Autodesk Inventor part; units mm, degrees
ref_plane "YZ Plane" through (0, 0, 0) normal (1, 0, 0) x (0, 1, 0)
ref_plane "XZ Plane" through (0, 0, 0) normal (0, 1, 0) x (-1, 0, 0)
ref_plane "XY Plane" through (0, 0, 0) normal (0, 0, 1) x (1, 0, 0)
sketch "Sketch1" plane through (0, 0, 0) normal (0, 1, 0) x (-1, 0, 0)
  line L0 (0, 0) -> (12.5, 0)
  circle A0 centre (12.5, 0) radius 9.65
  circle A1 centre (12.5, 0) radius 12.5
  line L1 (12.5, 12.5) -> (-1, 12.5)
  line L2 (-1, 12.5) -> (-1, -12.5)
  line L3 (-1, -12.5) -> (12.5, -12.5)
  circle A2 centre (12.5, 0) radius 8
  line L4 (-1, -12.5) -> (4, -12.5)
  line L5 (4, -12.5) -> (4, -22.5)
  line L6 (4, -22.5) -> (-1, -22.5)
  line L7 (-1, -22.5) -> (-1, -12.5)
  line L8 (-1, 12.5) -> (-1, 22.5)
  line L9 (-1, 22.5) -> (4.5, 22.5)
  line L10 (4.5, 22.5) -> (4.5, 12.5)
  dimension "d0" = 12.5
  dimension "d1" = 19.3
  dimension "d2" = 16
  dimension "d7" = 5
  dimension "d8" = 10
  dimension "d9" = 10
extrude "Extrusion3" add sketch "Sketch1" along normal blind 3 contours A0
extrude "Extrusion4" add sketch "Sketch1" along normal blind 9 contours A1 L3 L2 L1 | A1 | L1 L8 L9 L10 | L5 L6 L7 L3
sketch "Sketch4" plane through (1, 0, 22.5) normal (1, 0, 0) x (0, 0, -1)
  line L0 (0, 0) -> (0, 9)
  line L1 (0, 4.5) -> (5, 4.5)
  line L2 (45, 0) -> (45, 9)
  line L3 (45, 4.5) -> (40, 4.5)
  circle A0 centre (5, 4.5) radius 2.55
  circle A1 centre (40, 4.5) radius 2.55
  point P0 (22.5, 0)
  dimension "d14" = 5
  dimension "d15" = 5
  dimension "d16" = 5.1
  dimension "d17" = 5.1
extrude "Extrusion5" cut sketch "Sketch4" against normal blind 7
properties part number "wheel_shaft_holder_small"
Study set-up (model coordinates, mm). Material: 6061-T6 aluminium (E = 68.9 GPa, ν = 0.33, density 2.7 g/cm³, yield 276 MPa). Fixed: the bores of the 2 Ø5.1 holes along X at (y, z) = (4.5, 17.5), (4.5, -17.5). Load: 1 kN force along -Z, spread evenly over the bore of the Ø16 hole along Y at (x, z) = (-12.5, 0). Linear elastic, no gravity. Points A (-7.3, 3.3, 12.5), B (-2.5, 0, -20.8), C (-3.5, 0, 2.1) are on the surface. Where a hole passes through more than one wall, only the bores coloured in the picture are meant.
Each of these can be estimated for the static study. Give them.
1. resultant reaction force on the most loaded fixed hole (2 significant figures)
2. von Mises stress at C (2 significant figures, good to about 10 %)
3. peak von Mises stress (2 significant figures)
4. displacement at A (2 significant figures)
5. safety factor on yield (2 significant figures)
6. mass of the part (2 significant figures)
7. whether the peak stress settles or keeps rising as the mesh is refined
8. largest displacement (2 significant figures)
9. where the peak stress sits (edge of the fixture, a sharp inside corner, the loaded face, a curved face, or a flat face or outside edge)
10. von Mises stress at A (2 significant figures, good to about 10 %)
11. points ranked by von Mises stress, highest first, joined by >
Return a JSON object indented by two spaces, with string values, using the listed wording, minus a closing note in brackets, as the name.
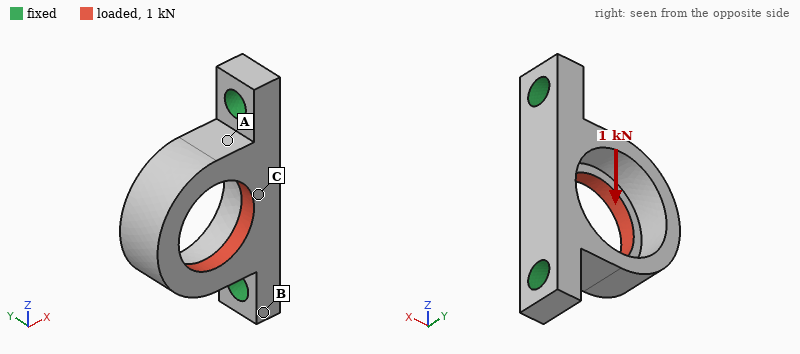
{
  "resultant reaction force on the most loaded fixed hole": "640 N",
  "von Mises stress at C": "28 MPa",
  "peak von Mises stress": "82 MPa",
  "displacement at A": "6.3 µm",
  "safety factor on yield": "3.4",
  "mass of the part": "9.8 g",
  "whether the peak stress settles or keeps rising as the mesh is refined": "settles",
  "largest displacement": "35 µm",
  "where the peak stress sits": "the loaded face",
  "von Mises stress at A": "48 MPa",
  "points ranked by von Mises stress, highest first, joined by >": "A > C > B"
}
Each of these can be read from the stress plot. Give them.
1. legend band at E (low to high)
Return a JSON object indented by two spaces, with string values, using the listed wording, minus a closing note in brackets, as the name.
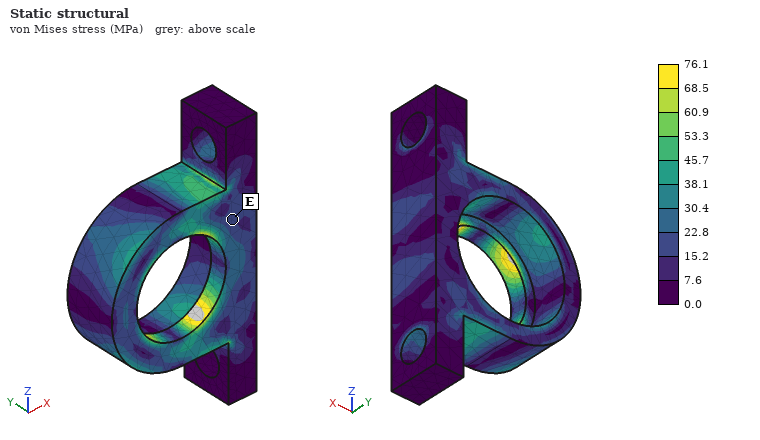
{
  "legend band at E": "15.2 to 22.8 MPa"
}
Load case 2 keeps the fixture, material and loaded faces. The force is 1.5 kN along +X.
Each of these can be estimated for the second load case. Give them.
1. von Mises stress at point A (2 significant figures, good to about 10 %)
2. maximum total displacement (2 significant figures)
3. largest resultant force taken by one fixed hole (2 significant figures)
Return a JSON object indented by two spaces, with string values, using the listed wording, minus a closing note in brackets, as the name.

{
  "von Mises stress at point A": "44 MPa",
  "maximum total displacement": "54 µm",
  "largest resultant force taken by one fixed hole": "770 N"
}
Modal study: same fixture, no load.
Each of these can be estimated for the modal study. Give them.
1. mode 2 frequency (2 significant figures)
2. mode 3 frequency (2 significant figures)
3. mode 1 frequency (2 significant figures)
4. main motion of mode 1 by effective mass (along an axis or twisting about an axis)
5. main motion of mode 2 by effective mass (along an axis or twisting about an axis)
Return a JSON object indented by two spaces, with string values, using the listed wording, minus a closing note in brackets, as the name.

{
  "mode 2 frequency": "12 kHz",
  "mode 3 frequency": "18 kHz",
  "mode 1 frequency": "7300 Hz",
  "main motion of mode 1 by effective mass": "along Y",
  "main motion of mode 2 by effective mass": "along Z"
}
